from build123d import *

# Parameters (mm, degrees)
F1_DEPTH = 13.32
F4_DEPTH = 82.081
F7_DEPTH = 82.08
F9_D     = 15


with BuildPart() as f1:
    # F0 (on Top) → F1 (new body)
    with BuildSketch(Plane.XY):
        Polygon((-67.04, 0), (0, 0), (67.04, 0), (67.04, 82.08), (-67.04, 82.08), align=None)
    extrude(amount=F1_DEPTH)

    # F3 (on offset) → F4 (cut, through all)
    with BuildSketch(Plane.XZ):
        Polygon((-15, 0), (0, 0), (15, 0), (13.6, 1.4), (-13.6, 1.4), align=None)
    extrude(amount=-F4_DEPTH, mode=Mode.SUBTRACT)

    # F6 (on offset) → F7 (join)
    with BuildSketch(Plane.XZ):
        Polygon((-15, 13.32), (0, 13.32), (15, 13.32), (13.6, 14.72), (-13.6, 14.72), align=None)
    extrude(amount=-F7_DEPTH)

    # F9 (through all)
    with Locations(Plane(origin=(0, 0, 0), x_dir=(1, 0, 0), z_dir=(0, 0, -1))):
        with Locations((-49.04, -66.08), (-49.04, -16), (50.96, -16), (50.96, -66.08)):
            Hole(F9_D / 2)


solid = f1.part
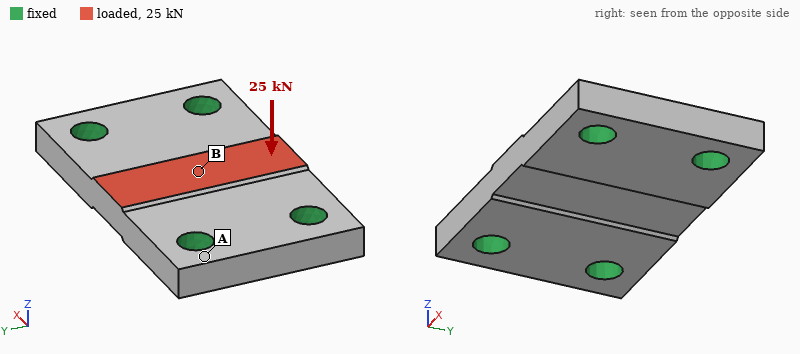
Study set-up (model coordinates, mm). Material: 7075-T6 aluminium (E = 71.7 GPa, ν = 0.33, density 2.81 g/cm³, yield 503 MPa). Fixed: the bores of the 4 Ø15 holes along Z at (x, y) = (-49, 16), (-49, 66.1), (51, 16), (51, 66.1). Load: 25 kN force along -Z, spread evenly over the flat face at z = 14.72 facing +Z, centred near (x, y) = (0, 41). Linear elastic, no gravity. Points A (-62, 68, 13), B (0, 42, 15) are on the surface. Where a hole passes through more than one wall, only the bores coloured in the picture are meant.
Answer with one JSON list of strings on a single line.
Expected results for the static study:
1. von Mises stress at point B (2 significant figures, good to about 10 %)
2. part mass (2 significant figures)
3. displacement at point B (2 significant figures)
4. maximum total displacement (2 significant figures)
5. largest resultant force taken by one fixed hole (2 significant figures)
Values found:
["72 MPa", "390 g", "0.096 mm", "0.11 mm", "7.0 kN"]
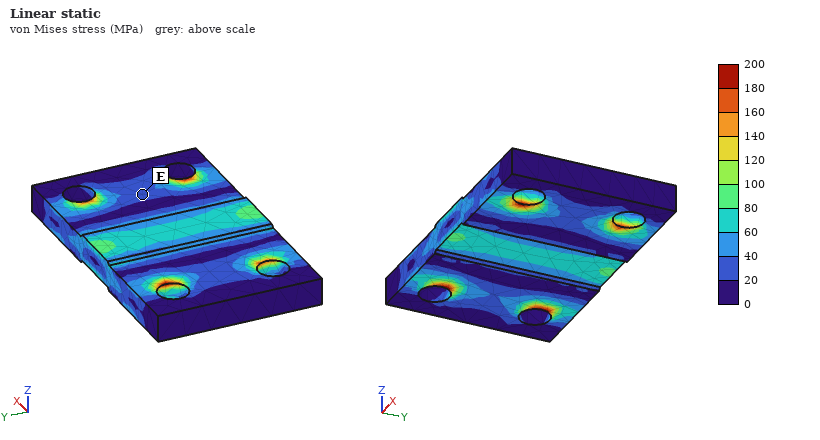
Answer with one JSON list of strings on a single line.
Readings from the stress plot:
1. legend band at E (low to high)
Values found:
["20 to 40 MPa"]
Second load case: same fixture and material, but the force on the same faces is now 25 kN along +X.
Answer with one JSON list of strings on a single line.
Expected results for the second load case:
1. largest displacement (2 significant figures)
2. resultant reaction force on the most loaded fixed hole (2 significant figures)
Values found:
["12 µm", "6.6 kN"]
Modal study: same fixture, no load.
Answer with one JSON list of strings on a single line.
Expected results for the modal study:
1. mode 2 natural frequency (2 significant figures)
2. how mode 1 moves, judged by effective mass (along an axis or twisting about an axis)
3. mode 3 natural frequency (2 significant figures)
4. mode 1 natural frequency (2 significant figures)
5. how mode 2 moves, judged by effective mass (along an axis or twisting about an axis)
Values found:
["8800 Hz", "along Z", "14 kHz", "7100 Hz", "twisting about X"]
